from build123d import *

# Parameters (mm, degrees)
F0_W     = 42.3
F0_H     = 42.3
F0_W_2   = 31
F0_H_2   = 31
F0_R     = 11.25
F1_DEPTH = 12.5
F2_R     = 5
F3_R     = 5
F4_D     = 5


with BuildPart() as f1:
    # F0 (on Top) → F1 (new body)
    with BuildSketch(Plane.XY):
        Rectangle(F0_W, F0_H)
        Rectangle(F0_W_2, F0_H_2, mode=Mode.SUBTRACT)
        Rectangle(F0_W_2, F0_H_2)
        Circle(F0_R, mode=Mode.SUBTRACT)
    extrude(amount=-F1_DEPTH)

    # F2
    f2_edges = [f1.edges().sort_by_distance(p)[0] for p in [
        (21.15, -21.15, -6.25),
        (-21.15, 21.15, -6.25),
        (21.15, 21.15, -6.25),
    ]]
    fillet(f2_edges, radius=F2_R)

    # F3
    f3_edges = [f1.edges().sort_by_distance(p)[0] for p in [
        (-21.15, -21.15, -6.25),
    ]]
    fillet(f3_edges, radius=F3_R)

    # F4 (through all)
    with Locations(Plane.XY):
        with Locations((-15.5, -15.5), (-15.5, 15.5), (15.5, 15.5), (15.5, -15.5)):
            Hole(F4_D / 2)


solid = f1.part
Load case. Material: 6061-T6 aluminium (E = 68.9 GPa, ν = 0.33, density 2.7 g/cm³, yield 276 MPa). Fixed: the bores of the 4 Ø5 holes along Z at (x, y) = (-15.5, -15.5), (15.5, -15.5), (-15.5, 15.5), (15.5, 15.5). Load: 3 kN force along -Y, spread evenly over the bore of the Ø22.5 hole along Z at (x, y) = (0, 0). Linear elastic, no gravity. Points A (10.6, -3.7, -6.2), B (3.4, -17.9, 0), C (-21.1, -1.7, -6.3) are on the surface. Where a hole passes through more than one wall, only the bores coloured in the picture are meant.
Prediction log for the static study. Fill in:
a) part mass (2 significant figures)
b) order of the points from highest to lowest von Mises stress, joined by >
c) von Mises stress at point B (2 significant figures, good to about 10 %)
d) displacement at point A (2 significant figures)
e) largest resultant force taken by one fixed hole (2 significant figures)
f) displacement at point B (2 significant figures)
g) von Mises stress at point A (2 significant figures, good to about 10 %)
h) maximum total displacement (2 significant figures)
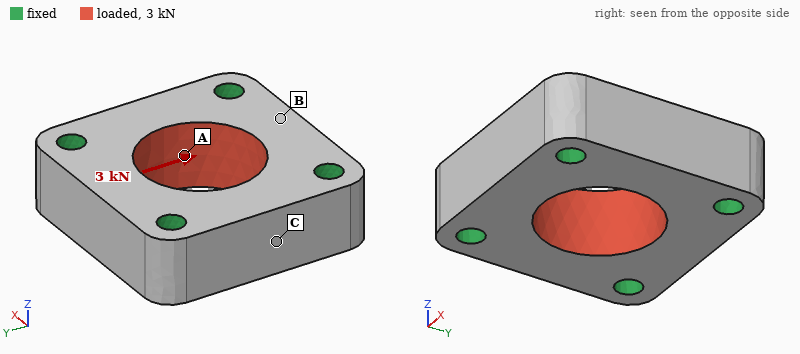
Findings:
44 g
A > B > C
3.4 MPa
0.87 µm
770 N
1.6 µm
6.4 MPa
2.0 µm
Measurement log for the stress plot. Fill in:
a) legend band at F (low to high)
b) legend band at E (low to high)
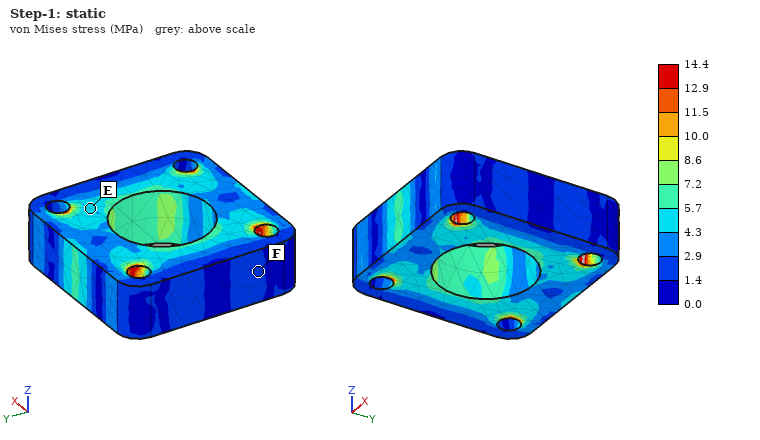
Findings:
1.4 to 2.9 MPa
4.3 to 5.7 MPa
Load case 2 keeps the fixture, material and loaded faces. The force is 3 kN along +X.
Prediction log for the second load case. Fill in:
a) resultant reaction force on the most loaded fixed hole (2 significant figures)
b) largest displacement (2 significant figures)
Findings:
770 N
2.0 µm
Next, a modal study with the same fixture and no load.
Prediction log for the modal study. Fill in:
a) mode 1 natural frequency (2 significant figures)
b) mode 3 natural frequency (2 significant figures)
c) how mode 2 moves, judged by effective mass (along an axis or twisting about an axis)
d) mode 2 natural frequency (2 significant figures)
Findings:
33 kHz
44 kHz
along Z
41 kHz
